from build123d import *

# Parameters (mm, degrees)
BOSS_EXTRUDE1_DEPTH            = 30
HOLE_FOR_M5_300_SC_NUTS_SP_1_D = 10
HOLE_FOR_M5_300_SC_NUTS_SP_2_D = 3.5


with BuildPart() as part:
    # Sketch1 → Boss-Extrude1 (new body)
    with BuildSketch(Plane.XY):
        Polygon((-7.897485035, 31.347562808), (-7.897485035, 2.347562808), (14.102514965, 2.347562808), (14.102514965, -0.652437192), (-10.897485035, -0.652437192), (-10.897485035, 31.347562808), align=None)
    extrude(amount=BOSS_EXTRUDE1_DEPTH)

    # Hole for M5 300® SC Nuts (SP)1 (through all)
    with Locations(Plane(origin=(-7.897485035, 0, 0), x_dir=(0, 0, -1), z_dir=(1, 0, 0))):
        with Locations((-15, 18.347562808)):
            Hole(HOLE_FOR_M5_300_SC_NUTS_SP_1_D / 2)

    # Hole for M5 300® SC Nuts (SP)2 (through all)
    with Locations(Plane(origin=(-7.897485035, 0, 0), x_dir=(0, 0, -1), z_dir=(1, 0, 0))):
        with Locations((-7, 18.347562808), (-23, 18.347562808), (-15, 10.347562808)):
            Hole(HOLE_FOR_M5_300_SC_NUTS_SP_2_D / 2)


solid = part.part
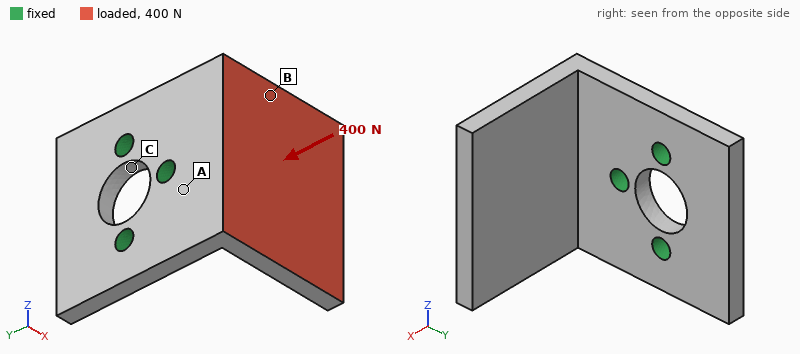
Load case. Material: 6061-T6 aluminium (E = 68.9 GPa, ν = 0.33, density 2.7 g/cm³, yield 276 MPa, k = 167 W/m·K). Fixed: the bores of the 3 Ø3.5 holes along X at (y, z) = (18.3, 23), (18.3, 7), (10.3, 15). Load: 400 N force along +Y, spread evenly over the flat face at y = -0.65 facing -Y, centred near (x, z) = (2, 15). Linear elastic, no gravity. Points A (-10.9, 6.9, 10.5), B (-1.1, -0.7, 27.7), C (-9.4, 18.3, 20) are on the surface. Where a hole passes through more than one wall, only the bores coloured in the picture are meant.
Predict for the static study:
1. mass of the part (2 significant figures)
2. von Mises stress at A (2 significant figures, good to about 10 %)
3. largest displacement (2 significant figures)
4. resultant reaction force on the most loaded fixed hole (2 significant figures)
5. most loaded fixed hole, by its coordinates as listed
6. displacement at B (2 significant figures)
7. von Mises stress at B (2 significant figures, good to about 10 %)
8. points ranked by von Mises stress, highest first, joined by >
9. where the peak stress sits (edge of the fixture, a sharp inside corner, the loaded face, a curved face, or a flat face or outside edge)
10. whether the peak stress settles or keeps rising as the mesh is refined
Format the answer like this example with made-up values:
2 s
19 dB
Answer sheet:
12 g
85 MPa
0.32 mm
340 N
(10.3, 15)
0.11 mm
41 MPa
A > B > C
edge of the fixture
keeps rising
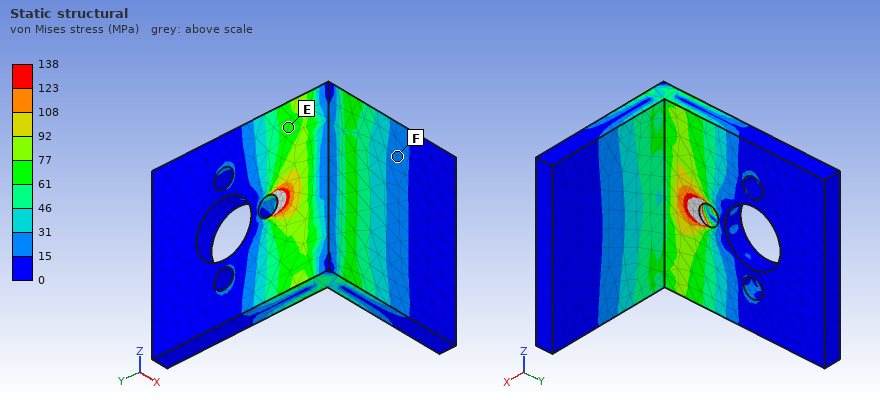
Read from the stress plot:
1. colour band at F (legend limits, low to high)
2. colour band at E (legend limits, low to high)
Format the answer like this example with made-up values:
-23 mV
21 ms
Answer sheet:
15 to 31 MPa
61 to 77 MPa
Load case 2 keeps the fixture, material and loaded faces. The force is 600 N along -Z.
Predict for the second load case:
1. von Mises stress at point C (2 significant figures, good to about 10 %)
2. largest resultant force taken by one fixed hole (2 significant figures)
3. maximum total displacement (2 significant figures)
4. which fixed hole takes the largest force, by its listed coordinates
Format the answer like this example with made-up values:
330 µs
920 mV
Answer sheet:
28 MPa
640 N
0.18 mm
(10.3, 15)
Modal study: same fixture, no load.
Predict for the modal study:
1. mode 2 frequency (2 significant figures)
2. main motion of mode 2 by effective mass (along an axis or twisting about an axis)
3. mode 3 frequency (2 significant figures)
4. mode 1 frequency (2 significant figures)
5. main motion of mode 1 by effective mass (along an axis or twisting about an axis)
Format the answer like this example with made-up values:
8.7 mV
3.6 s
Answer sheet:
3900 Hz
along Z
8000 Hz
2700 Hz
along Y
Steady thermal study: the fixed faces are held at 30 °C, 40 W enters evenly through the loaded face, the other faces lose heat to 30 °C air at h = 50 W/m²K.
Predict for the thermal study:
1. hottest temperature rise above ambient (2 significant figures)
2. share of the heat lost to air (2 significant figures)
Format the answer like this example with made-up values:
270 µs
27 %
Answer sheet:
55 K
7.1 %
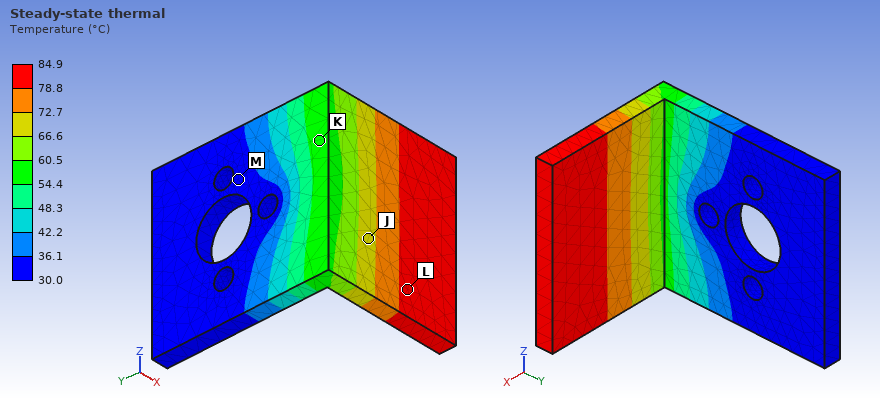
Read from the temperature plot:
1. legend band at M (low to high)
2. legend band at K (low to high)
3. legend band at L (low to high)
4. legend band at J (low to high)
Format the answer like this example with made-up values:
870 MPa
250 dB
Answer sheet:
30.0 to 36.1 °C
54.4 to 60.5 °C
78.8 to 84.9 °C
66.6 to 72.7 °C
